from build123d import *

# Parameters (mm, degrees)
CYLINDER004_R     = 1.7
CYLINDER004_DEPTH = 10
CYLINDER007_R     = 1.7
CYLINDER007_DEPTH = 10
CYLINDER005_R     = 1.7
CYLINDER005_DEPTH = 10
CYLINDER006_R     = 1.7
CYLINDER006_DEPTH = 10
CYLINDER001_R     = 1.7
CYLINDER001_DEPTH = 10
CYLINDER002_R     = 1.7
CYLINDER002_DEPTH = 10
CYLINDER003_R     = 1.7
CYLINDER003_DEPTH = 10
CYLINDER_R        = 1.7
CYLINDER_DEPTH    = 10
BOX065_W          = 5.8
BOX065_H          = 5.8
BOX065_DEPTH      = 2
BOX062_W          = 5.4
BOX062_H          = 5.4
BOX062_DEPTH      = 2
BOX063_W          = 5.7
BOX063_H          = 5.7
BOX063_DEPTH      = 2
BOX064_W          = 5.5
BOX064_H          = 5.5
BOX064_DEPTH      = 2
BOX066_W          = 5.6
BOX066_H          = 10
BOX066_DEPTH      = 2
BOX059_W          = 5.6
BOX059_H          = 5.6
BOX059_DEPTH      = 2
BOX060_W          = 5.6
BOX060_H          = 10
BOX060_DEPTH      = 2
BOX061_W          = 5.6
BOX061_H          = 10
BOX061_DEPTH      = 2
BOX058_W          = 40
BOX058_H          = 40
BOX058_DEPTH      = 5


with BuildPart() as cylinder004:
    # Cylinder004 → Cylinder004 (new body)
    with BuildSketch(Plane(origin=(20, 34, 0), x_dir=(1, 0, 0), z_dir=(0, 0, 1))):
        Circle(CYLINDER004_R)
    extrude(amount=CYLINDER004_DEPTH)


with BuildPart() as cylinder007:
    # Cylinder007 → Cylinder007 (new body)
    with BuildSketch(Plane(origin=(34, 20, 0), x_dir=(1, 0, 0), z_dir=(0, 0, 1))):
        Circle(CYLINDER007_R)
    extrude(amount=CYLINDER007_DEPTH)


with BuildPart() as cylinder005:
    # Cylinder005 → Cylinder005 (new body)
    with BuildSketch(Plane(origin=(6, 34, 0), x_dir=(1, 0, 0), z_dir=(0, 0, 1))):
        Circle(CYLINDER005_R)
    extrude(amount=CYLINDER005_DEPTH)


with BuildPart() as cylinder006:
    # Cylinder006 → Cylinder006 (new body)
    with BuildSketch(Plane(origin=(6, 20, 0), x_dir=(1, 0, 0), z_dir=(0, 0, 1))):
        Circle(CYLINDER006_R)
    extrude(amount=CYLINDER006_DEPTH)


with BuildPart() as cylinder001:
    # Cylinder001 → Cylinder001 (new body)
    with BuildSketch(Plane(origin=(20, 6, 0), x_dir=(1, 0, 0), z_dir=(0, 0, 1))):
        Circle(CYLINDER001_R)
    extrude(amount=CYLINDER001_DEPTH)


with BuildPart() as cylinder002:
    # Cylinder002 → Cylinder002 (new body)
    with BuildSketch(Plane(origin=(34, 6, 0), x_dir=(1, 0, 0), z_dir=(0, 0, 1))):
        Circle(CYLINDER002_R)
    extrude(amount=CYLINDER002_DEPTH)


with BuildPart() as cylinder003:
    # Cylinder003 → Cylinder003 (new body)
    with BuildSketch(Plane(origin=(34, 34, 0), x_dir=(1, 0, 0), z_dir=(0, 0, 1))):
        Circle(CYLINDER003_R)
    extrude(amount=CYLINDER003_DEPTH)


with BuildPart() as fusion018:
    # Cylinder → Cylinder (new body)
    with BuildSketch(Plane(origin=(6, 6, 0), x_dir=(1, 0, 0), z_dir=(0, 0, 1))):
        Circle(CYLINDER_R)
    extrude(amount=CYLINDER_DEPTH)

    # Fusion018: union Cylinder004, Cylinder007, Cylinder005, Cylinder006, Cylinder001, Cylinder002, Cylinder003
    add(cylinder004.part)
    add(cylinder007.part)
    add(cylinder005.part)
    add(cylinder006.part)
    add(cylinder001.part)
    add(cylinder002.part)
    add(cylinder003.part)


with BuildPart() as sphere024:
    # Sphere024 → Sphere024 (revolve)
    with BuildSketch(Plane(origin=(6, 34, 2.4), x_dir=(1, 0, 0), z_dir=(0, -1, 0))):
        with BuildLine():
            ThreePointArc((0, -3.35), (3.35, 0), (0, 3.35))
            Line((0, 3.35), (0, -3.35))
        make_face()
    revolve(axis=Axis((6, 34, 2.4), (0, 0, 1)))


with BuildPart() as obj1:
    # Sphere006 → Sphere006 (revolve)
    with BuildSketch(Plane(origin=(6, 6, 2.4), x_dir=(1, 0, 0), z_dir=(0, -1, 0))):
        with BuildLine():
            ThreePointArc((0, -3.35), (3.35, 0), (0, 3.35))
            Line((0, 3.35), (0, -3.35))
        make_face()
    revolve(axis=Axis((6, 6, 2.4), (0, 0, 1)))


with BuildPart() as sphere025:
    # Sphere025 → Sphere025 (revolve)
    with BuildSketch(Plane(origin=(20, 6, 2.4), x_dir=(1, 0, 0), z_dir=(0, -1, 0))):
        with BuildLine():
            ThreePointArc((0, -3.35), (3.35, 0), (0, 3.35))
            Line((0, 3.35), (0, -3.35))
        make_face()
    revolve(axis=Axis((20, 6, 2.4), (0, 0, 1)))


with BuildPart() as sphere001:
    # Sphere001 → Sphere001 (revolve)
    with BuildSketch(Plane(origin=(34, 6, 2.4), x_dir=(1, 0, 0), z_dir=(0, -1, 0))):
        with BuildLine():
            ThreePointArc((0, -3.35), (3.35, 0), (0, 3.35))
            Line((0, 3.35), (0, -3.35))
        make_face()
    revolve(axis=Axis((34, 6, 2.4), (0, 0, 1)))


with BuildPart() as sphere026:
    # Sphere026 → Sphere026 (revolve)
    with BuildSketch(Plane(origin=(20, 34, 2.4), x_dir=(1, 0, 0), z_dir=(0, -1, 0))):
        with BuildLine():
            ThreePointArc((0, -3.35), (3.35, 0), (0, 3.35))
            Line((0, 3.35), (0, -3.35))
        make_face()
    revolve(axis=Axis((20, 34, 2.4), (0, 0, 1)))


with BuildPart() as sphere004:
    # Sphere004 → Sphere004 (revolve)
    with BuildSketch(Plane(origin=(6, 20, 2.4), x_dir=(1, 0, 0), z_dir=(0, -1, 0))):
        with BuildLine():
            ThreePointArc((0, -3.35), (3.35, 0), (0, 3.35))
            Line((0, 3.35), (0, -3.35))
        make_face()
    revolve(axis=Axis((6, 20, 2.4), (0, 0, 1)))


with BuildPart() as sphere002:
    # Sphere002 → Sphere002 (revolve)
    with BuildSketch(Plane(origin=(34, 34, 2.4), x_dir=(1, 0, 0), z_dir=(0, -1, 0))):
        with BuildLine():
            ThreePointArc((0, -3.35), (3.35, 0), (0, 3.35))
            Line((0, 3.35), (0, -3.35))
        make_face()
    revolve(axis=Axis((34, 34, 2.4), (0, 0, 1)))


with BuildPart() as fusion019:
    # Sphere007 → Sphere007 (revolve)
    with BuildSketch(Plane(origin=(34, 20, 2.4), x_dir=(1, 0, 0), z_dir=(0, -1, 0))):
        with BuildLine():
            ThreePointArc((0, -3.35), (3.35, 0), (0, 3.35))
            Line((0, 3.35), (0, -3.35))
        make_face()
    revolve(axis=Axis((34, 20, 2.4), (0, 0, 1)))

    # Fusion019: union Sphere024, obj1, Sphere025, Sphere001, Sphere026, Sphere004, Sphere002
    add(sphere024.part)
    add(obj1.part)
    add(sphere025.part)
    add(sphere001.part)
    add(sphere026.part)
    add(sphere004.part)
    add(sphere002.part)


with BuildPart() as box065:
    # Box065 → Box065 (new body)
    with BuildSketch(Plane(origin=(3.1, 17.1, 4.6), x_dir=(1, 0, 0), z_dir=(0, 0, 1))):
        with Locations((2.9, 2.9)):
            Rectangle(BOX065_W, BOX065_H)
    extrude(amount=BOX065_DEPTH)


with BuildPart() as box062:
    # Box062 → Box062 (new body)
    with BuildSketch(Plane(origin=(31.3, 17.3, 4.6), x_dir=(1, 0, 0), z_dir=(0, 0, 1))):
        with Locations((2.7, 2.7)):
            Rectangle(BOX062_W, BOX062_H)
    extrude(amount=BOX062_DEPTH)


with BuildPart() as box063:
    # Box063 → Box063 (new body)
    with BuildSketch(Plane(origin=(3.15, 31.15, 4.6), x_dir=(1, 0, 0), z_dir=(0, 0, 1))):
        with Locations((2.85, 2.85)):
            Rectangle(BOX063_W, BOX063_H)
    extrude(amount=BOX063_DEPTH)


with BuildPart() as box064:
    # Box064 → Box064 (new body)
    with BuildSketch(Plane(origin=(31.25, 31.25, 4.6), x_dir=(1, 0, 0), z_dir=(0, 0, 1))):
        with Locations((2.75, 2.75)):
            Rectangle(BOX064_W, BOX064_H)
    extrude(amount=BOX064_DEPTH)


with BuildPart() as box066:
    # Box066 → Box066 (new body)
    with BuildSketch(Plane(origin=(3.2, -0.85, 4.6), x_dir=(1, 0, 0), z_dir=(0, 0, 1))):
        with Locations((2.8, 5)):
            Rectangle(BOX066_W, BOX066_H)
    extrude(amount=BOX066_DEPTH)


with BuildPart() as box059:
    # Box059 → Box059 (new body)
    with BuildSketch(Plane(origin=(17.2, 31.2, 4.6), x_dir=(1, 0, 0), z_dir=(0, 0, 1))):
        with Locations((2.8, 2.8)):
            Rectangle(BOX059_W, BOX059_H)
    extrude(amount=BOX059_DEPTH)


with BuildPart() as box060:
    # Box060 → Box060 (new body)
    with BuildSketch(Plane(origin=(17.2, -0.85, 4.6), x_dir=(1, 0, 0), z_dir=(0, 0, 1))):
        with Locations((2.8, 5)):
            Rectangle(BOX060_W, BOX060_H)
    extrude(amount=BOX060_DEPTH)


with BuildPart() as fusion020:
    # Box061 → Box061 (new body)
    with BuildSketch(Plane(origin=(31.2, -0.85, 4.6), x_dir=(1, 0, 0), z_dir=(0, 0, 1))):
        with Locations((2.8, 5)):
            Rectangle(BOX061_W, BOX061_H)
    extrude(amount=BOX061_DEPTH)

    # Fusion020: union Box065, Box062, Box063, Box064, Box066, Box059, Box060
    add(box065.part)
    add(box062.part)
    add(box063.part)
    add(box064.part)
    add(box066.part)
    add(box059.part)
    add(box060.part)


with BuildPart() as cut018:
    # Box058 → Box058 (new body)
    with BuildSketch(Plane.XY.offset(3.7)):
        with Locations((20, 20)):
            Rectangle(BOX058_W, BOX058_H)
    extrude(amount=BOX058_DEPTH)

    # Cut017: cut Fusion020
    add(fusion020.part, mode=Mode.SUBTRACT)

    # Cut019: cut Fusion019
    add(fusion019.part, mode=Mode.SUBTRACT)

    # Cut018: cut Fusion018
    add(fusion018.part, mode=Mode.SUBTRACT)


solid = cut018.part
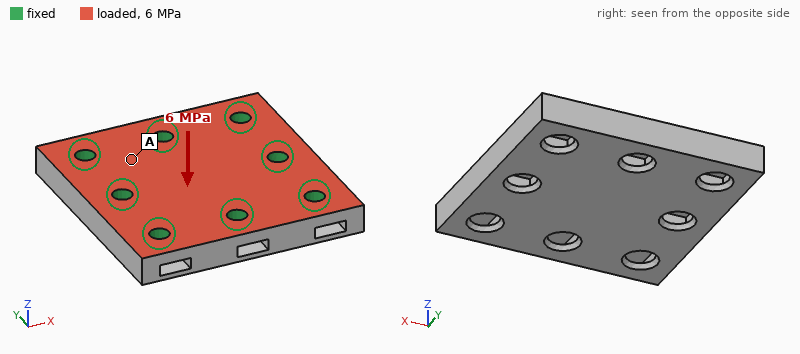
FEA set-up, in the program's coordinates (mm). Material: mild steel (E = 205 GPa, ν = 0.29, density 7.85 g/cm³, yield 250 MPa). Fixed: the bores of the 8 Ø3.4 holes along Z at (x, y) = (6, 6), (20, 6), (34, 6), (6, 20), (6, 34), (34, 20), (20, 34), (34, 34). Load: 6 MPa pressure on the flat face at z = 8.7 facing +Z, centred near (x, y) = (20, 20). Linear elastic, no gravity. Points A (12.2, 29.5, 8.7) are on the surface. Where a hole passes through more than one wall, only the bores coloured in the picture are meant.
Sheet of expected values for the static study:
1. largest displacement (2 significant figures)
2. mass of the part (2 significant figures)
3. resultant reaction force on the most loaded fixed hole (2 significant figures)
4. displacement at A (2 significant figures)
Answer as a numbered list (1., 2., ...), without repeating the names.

1. 4.6 µm
2. 55 g
3. 1.3 kN
4. 2.4 µm
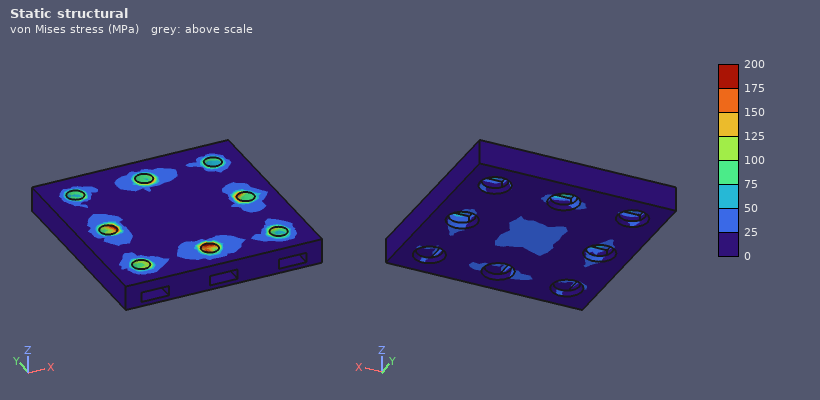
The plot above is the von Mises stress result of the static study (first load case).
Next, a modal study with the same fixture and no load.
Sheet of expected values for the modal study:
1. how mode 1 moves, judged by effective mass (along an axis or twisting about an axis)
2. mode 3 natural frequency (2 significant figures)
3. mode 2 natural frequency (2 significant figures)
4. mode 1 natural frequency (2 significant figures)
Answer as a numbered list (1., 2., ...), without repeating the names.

1. along Z
2. 47 kHz
3. 46 kHz
4. 33 kHz
